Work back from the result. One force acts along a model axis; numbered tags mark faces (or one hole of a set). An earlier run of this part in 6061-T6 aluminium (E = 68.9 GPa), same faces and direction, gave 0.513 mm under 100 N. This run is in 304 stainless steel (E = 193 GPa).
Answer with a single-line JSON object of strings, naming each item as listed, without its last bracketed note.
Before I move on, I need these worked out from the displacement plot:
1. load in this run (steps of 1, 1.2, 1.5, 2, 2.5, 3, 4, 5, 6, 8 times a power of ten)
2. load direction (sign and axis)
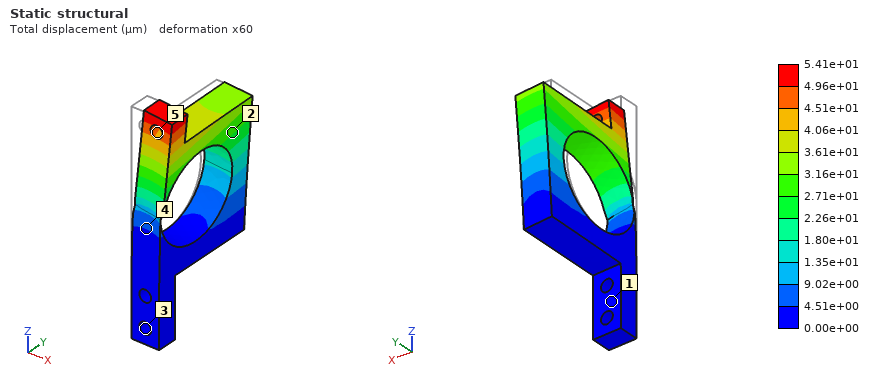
{"load in this run": "30 N", "load direction": "+X"}
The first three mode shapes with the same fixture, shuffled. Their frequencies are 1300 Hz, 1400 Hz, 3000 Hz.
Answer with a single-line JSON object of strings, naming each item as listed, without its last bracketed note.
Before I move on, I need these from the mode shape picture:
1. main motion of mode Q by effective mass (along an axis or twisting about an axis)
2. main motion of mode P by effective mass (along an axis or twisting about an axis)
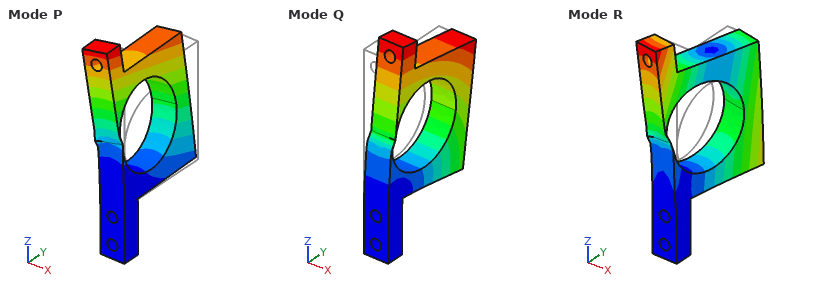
{"main motion of mode Q by effective mass": "along Y", "main motion of mode P by effective mass": "along X"}
